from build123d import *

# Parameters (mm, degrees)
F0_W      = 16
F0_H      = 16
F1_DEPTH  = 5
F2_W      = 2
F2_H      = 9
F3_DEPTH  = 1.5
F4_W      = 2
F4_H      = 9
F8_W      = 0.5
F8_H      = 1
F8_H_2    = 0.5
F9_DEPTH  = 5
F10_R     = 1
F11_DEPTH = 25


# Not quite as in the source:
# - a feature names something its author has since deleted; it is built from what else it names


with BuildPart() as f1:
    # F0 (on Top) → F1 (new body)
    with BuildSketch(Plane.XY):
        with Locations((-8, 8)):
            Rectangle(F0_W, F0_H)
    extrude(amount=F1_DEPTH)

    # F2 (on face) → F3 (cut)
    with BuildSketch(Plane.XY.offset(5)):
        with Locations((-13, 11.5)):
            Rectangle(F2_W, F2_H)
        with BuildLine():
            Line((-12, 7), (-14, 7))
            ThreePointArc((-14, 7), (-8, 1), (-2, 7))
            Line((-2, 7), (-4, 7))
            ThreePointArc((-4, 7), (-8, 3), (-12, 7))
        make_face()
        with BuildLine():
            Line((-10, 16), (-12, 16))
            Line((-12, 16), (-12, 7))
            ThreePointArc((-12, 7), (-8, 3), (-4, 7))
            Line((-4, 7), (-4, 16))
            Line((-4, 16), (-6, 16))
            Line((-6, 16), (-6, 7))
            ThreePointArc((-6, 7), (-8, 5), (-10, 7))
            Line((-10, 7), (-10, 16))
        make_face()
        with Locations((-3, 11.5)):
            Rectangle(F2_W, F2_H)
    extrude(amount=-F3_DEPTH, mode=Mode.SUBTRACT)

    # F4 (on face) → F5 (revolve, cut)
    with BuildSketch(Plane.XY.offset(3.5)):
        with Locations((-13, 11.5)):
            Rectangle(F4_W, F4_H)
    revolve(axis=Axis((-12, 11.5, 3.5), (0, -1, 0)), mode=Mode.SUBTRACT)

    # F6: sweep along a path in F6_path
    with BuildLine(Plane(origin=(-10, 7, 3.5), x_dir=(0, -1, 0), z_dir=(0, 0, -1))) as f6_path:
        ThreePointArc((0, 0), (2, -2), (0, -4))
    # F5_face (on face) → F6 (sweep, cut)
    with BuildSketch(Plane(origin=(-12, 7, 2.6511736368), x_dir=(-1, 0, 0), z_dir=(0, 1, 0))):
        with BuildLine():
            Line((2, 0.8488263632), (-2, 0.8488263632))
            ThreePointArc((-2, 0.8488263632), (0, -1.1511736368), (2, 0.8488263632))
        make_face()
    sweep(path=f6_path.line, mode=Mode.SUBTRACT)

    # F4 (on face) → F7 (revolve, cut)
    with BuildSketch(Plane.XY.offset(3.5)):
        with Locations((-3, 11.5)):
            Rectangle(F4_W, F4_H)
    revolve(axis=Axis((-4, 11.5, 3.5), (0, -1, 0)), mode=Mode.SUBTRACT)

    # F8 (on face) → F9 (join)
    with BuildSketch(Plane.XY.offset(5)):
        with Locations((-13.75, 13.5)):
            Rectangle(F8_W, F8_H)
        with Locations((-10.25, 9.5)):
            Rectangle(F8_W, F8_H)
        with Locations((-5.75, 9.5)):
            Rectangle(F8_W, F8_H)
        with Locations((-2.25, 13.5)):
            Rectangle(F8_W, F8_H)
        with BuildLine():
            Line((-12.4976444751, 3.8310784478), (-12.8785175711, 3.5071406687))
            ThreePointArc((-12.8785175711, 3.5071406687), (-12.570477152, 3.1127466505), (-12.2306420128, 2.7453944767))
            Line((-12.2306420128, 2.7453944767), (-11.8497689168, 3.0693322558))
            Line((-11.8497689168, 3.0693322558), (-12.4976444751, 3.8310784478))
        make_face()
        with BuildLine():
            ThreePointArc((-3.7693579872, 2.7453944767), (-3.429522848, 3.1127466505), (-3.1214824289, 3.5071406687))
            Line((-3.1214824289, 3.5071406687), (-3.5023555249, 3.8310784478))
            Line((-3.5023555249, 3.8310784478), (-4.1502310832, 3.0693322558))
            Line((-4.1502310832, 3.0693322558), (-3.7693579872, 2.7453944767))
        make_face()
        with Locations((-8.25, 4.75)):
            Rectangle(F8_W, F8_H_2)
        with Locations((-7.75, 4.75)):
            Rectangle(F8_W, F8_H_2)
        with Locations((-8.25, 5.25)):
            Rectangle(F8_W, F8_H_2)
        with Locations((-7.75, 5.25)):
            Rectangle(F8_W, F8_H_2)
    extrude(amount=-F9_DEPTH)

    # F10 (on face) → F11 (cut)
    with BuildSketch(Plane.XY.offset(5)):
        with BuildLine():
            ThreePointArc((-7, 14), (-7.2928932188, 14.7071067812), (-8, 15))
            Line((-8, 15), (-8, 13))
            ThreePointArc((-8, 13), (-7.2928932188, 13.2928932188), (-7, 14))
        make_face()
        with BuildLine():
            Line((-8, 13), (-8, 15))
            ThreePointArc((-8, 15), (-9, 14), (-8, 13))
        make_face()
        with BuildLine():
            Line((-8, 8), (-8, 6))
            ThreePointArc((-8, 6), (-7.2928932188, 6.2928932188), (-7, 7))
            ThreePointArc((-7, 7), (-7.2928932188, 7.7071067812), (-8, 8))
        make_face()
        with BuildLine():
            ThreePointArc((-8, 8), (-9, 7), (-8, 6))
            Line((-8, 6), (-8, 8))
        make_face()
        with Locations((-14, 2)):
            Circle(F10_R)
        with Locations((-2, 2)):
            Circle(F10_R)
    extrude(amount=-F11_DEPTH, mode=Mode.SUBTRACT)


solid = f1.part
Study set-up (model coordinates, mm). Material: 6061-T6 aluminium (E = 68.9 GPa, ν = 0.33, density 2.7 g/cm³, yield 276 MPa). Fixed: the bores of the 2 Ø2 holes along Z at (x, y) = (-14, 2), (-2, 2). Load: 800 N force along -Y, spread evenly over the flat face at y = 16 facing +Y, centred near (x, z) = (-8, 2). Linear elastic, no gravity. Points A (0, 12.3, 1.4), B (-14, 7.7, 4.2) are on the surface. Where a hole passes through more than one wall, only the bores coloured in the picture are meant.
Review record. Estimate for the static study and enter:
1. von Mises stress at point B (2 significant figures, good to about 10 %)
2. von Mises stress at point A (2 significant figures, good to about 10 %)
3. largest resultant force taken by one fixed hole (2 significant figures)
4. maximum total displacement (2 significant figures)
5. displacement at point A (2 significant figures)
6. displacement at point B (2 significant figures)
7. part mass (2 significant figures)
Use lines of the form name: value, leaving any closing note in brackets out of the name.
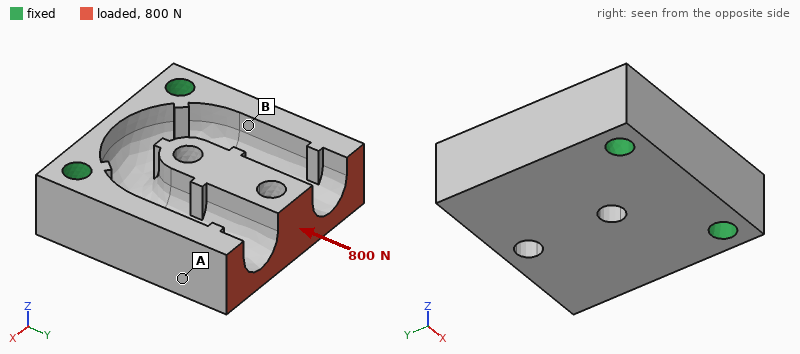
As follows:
von Mises stress at point B: 27 MPa
von Mises stress at point A: 14 MPa
largest resultant force taken by one fixed hole: 400 N
maximum total displacement: 11 µm
displacement at point A: 2.7 µm
displacement at point B: 2.2 µm
part mass: 2.3 g
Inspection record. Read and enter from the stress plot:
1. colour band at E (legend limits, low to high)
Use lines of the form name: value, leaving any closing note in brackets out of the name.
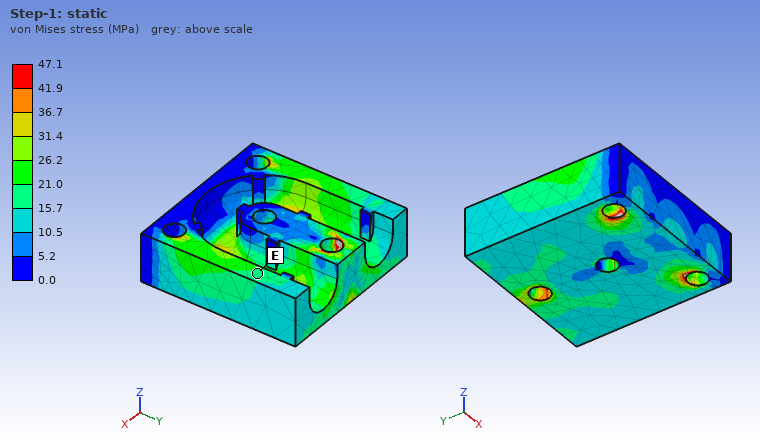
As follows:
colour band at E: 15.7 to 21.0 MPa
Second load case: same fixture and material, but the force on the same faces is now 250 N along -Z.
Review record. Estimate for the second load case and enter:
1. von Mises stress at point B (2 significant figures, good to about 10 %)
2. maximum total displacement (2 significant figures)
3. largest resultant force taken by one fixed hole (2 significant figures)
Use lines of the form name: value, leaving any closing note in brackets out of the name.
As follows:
von Mises stress at point B: 84 MPa
maximum total displacement: 61 µm
largest resultant force taken by one fixed hole: 130 N
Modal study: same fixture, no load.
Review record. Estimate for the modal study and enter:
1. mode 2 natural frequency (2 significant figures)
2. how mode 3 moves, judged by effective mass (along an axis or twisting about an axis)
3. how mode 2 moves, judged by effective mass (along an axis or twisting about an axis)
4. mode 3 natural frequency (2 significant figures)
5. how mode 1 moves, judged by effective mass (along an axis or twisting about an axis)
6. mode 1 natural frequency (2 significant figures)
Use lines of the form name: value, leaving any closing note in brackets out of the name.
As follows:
mode 2 natural frequency: 24 kHz
how mode 3 moves, judged by effective mass: along X
how mode 2 moves, judged by effective mass: along X
mode 3 natural frequency: 37 kHz
how mode 1 moves, judged by effective mass: along Z
mode 1 natural frequency: 15 kHz
